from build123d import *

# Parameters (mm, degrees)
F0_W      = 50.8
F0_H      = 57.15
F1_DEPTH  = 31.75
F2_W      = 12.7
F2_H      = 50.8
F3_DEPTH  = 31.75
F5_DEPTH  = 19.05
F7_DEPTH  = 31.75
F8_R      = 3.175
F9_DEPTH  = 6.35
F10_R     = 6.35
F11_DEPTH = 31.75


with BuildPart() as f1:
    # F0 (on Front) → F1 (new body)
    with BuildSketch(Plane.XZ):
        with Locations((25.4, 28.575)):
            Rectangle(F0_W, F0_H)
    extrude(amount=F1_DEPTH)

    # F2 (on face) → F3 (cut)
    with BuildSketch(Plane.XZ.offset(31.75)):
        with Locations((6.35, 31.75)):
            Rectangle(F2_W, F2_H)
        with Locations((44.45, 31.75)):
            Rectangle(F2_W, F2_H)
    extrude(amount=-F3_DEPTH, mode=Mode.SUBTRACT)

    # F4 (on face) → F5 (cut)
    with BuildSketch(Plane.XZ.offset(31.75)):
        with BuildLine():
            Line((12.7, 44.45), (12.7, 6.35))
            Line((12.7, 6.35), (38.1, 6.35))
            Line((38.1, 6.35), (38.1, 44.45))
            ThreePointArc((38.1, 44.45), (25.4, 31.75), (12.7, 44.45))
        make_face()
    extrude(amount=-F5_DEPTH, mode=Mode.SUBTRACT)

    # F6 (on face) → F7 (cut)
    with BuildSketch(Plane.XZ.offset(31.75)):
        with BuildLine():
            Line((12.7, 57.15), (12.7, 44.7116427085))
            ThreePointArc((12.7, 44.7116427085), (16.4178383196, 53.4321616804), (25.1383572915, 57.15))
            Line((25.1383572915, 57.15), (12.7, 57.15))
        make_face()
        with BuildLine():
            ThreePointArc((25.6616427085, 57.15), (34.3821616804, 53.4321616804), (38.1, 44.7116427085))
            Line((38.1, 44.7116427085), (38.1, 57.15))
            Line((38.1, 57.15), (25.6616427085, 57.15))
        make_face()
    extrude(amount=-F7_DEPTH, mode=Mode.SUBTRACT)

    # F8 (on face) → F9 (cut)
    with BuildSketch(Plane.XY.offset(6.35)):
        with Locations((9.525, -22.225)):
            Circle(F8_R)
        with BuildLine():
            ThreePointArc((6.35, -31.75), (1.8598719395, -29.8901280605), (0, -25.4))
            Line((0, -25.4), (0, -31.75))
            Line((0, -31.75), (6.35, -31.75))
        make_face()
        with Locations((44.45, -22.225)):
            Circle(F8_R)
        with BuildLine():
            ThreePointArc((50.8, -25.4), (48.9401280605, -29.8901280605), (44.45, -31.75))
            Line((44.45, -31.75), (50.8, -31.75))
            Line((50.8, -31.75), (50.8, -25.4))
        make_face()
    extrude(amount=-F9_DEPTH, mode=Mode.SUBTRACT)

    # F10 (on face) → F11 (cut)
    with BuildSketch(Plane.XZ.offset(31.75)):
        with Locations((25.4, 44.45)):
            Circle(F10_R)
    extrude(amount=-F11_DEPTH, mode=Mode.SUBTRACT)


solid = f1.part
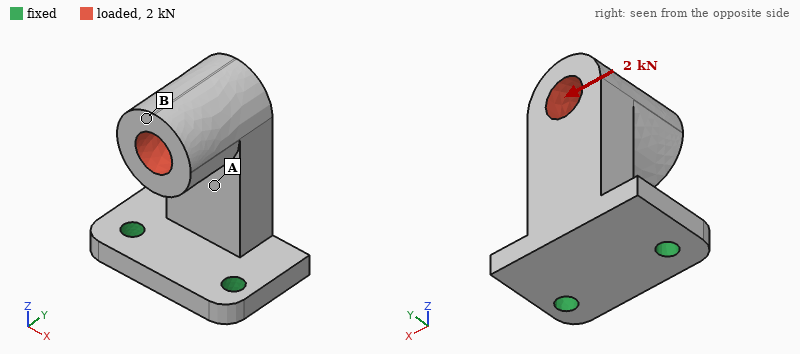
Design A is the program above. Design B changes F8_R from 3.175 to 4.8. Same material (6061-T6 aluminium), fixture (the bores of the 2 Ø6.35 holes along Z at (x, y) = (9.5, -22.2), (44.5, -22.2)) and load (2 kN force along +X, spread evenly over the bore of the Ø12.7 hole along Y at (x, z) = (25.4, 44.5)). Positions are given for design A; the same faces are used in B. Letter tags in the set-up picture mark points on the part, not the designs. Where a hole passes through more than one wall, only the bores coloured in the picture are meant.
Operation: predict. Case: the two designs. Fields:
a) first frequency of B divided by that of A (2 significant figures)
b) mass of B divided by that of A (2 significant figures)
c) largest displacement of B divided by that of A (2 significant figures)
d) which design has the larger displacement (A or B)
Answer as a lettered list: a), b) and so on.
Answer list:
a) 1.1
b) 0.98
c) 0.88
d) A
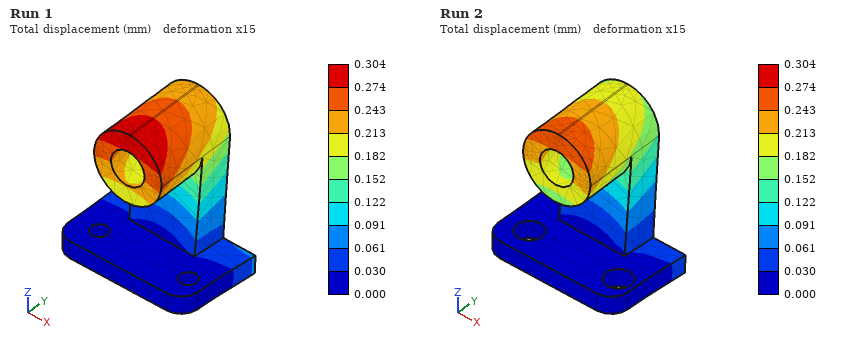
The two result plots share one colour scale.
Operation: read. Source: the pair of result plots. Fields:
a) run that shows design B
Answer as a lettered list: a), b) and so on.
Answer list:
a) Run 2
